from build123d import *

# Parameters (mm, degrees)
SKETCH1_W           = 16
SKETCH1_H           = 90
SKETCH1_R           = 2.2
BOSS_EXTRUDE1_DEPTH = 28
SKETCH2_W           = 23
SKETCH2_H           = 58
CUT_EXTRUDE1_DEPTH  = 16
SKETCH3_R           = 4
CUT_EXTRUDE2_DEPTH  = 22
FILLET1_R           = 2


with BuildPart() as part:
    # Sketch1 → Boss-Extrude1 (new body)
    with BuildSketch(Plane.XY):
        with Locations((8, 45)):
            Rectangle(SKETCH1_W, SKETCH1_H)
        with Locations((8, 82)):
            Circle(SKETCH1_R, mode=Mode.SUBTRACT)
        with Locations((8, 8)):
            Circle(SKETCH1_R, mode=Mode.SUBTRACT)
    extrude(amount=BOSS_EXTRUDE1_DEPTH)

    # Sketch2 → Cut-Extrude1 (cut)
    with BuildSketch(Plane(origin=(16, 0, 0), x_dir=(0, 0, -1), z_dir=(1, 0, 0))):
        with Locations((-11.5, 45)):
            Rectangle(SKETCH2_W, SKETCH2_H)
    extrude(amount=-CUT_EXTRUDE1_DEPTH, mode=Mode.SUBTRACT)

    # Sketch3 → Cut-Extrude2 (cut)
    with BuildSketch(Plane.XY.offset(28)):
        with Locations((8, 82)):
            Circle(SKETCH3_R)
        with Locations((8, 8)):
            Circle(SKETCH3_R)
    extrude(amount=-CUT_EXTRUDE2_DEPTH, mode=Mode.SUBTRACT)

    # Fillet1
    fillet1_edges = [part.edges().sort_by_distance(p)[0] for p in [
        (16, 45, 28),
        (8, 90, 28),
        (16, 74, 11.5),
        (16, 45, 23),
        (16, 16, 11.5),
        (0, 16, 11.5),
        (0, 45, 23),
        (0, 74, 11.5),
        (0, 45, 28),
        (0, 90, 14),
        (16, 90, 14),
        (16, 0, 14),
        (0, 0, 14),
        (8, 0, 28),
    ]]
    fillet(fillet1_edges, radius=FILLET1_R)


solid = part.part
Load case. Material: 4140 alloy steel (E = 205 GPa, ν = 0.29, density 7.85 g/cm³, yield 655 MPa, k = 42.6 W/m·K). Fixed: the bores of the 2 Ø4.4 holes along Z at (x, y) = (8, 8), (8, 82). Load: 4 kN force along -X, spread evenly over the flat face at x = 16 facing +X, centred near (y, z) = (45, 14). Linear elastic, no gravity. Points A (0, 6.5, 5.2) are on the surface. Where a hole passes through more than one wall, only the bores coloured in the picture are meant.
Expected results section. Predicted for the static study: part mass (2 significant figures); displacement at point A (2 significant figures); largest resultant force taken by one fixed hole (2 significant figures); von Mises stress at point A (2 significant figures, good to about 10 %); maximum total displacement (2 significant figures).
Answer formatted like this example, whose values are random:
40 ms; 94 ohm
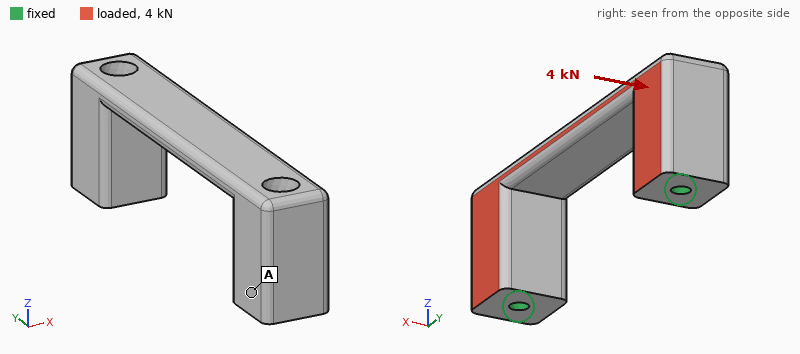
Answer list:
130 g; 5.7 µm; 2.0 kN; 33 MPa; 26 µm
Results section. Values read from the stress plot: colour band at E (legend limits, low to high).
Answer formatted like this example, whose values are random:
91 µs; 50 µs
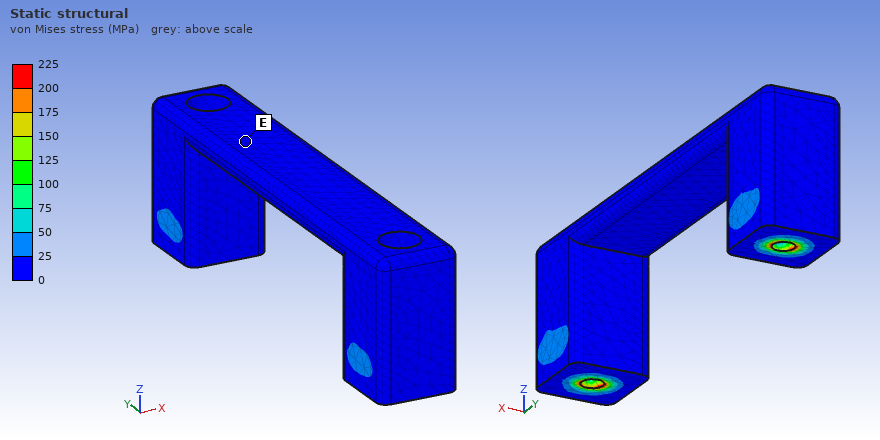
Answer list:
0 to 25 MPa
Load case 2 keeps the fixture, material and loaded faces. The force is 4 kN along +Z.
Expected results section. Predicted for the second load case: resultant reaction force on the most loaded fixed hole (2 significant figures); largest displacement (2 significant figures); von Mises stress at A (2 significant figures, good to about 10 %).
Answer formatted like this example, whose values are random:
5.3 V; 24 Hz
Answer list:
2.0 kN; 24 µm; 20 MPa
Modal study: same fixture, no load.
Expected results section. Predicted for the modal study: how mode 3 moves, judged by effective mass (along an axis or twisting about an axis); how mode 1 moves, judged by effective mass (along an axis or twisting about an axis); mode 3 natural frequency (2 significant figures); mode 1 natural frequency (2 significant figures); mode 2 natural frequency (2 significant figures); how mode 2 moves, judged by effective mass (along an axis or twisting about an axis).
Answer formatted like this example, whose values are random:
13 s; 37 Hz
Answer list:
along Y; along X; 6200 Hz; 5300 Hz; 5900 Hz; along Z
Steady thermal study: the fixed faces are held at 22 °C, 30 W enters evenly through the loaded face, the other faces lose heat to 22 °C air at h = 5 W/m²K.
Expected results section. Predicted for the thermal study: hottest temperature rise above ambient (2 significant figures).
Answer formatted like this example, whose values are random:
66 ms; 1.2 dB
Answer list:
33 K
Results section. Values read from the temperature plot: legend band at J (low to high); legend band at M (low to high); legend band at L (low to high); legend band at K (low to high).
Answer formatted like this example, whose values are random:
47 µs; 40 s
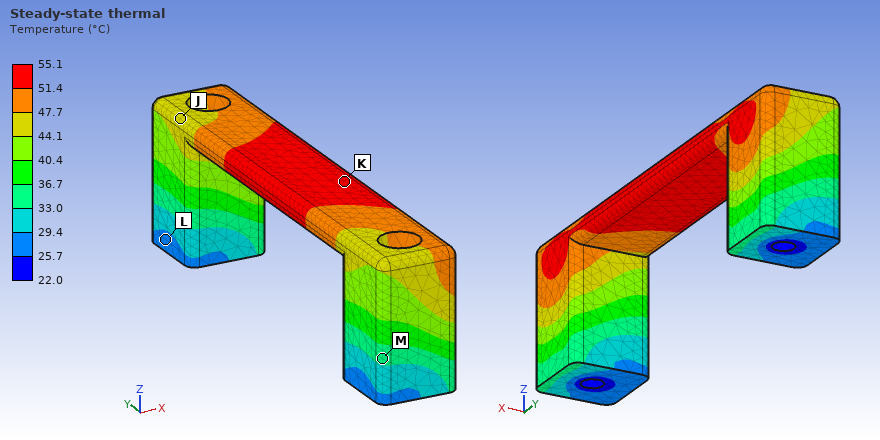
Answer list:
44.1 to 47.7 °C; 33.0 to 36.7 °C; 25.7 to 29.4 °C; 51.4 to 55.1 °C
